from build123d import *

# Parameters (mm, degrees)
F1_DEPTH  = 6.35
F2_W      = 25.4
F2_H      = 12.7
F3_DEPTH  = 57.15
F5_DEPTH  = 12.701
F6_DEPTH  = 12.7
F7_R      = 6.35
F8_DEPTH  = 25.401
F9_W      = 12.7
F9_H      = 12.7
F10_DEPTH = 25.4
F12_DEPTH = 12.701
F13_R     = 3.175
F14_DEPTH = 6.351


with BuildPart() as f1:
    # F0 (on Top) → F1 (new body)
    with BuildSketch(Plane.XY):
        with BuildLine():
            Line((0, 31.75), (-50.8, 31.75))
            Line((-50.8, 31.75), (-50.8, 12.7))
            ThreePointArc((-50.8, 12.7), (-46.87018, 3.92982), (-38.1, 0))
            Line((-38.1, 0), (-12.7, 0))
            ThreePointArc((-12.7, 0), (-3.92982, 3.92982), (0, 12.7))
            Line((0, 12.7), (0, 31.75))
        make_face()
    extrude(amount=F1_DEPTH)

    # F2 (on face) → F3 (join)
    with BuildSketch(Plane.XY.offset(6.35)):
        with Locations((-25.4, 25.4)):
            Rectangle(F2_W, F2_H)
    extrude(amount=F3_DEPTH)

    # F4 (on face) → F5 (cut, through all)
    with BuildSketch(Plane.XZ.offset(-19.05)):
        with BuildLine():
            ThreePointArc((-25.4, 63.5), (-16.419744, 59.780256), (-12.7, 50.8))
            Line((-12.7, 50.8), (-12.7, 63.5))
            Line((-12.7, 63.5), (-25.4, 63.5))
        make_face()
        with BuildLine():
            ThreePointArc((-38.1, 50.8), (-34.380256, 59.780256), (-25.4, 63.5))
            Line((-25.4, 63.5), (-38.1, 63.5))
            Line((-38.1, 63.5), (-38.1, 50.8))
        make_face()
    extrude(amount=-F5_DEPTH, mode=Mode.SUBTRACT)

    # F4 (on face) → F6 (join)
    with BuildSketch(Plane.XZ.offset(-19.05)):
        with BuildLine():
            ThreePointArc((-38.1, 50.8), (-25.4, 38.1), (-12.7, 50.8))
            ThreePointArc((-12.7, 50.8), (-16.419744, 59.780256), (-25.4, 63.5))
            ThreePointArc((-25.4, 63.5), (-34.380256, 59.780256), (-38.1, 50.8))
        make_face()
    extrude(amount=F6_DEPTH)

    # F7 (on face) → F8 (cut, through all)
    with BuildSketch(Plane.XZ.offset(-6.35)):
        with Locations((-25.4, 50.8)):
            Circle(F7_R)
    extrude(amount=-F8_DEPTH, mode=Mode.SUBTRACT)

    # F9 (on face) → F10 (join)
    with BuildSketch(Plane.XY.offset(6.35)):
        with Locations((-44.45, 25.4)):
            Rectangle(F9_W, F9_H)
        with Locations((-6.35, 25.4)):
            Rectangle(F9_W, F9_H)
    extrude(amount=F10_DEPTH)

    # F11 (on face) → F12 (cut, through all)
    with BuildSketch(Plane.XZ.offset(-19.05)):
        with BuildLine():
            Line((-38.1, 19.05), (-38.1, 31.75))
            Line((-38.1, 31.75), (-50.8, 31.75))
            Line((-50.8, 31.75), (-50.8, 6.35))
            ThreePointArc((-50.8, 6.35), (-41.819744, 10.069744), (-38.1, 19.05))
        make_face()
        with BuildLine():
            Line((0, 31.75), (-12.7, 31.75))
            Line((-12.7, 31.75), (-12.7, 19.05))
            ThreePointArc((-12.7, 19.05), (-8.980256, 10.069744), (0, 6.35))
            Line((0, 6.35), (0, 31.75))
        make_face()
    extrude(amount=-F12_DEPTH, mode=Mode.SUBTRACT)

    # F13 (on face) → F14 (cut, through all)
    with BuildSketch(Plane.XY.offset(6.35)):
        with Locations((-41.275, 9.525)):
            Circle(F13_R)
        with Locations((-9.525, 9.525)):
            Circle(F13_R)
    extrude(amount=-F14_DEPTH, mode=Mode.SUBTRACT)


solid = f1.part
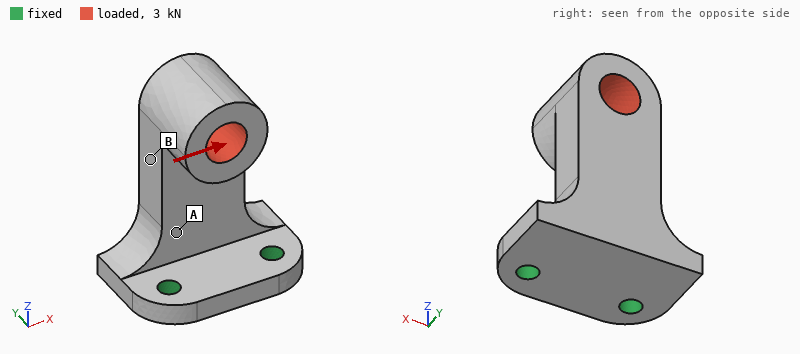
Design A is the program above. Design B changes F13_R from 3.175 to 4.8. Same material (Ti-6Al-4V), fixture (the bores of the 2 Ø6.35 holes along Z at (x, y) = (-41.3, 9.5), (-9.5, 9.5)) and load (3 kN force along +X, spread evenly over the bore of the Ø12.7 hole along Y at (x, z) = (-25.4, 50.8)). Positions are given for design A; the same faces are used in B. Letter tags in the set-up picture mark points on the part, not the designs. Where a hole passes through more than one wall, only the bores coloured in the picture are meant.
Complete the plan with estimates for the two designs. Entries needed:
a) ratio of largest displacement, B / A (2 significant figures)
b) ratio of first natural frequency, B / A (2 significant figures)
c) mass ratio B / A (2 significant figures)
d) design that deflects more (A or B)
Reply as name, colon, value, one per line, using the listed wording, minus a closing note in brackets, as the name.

ratio of largest displacement, B / A: 0.85
ratio of first natural frequency, B / A: 1.1
mass ratio B / A: 0.98
design that deflects more: A
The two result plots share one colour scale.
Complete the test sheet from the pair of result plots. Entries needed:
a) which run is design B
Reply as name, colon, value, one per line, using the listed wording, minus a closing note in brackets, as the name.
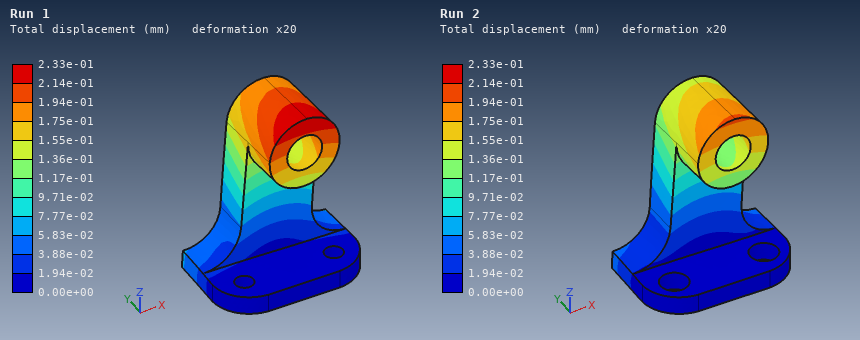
which run is design B: Run 2
